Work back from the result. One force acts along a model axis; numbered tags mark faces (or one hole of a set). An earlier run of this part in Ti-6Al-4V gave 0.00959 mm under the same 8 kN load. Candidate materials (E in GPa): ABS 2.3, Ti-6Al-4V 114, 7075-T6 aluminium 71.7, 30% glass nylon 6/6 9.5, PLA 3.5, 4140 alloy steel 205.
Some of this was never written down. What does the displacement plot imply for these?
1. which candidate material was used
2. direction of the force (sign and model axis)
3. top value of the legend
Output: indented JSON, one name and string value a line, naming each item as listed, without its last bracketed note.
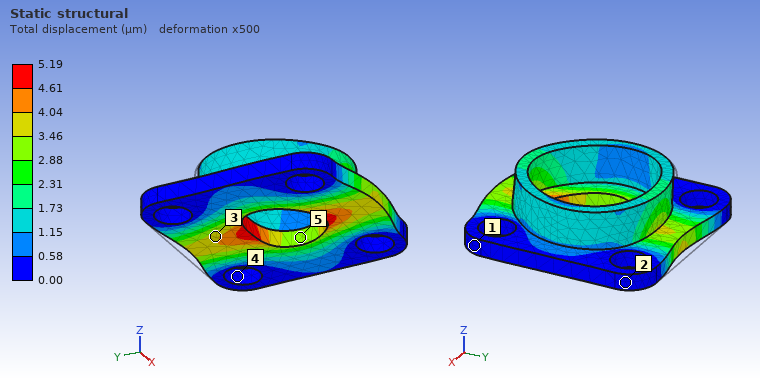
{
  "which candidate material was used": "4140 alloy steel",
  "direction of the force": "-Y",
  "top value of the legend": "5.19 µm"
}
